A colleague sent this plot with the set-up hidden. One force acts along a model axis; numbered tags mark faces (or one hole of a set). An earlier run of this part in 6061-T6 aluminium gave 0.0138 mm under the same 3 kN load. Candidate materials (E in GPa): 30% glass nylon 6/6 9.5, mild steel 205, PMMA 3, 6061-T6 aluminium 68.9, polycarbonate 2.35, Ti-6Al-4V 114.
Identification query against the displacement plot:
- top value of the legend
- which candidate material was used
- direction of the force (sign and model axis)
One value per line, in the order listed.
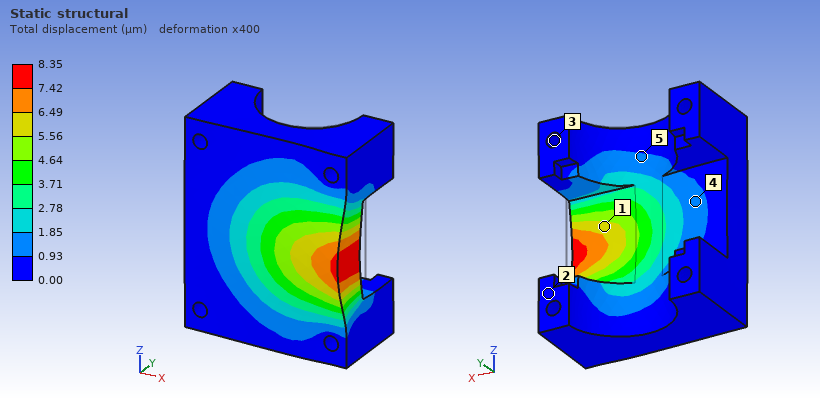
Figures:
8.35 µm
Ti-6Al-4V
-Y
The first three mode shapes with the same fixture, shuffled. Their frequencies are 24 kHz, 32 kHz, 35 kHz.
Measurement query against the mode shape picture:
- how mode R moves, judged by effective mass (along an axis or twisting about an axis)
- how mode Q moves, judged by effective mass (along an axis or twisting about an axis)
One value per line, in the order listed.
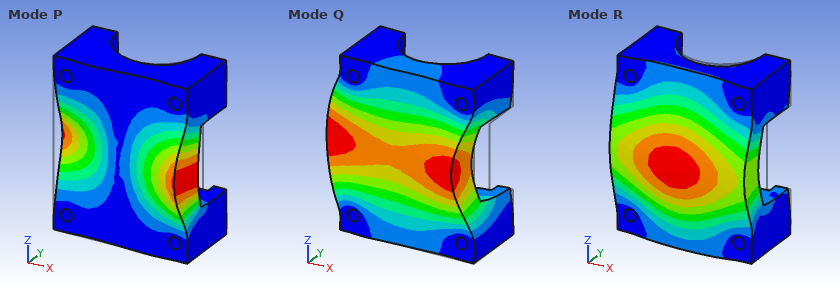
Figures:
along Y
along X
